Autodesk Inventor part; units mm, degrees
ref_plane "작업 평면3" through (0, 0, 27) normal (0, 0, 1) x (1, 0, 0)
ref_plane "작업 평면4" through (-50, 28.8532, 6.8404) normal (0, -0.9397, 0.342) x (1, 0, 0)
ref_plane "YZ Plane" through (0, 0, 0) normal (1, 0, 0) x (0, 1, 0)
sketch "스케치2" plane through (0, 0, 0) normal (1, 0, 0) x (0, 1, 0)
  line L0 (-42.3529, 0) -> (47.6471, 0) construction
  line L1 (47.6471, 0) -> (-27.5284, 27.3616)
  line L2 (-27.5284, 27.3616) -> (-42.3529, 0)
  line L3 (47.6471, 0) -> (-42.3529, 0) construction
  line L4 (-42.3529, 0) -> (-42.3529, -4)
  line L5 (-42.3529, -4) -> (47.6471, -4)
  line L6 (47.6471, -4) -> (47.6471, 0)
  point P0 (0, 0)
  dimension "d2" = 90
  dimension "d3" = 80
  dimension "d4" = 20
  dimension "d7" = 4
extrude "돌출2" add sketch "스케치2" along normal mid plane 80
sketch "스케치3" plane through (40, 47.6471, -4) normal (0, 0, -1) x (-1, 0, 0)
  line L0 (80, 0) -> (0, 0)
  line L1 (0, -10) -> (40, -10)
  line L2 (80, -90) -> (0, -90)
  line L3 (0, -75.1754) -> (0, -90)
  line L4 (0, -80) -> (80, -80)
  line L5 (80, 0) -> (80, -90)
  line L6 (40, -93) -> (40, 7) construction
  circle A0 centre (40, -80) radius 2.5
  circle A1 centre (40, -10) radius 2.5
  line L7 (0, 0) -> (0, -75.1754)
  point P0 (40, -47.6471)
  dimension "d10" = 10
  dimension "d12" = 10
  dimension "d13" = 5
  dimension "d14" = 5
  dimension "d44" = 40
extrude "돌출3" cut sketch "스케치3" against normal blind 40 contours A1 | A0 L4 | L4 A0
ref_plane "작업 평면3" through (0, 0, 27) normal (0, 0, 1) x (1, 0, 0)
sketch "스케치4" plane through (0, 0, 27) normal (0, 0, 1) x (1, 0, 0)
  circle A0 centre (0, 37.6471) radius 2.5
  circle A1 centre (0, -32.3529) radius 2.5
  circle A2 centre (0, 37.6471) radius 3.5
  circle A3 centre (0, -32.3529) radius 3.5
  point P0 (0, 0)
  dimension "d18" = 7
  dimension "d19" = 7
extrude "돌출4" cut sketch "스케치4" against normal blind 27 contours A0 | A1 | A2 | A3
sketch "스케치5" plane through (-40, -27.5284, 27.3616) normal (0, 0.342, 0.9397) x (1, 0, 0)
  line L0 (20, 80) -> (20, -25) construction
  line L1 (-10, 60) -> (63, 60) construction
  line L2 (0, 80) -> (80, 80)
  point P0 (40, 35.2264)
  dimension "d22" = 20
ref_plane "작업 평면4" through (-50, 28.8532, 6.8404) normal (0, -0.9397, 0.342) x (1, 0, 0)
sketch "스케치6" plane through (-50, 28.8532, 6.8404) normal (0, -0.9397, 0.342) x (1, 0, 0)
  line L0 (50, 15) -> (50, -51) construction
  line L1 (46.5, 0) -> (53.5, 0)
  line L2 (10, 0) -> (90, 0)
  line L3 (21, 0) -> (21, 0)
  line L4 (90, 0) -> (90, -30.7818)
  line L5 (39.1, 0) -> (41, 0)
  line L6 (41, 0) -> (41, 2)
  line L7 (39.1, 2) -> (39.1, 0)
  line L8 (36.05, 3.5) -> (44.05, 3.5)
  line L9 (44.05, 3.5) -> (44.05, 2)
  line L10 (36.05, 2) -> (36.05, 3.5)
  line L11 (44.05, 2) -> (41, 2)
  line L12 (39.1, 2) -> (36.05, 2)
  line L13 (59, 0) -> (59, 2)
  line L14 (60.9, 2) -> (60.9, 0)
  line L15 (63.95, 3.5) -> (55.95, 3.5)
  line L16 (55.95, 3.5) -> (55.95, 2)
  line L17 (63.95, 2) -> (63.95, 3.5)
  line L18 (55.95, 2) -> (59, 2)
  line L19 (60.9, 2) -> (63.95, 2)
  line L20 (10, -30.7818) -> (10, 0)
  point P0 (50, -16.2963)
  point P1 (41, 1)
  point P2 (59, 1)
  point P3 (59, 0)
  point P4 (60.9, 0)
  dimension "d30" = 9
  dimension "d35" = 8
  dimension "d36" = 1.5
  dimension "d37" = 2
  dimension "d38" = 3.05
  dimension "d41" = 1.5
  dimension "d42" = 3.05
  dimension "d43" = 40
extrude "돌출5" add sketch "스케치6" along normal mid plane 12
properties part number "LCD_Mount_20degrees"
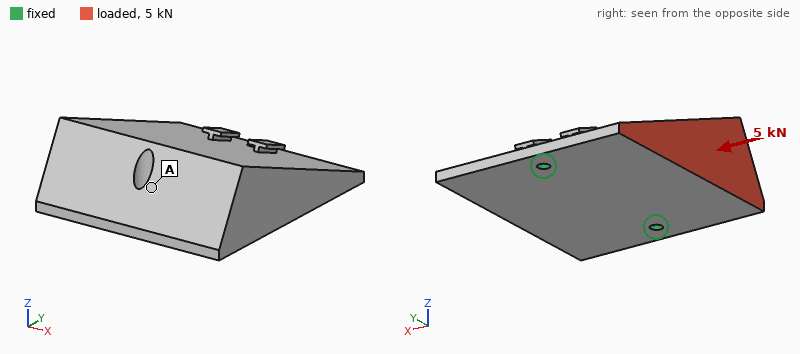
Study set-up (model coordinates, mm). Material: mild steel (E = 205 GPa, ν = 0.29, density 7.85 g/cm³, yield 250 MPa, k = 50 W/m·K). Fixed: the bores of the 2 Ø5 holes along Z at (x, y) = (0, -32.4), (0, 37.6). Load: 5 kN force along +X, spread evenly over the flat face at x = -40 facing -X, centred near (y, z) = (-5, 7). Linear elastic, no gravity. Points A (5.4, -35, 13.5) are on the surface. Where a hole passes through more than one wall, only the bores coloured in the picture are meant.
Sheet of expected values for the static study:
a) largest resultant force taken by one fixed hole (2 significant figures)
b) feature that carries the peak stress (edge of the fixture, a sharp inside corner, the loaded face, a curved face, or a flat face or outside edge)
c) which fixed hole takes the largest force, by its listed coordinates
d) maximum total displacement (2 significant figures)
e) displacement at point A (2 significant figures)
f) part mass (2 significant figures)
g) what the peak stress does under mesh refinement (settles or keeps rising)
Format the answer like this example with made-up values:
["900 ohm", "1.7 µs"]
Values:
["3.0 kN", "edge of the fixture", "(0, -32.4)", "69 µm", "24 µm", "990 g", "keeps rising"]
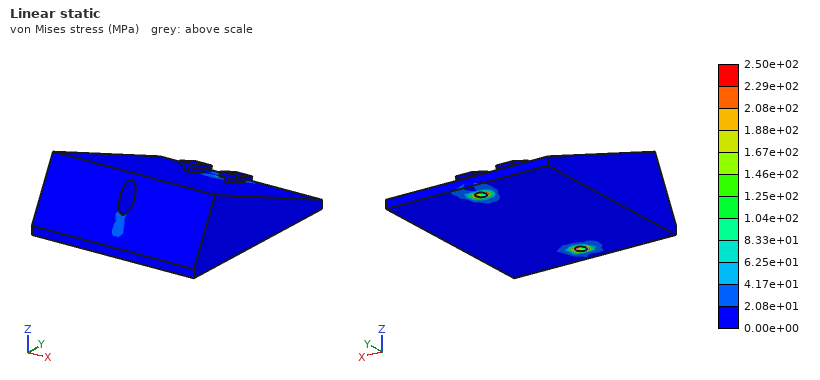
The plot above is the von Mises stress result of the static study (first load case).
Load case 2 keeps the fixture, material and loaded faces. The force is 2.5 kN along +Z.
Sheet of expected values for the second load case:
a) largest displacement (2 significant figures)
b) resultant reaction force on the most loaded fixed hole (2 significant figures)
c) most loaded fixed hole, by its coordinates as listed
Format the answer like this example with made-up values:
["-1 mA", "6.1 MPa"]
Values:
["0.16 mm", "1.8 kN", "(0, -32.4)"]
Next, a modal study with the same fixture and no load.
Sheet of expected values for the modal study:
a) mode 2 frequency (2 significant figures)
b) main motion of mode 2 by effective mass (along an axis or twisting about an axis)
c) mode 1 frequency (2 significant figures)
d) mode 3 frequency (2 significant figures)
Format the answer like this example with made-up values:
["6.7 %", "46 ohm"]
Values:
["5000 Hz", "along Z", "1100 Hz", "8000 Hz"]
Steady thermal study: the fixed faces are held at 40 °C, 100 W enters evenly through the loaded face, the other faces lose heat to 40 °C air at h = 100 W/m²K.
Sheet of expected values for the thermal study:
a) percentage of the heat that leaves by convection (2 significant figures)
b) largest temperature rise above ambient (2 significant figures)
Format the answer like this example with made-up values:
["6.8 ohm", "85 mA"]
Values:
["55 %", "67 K"]
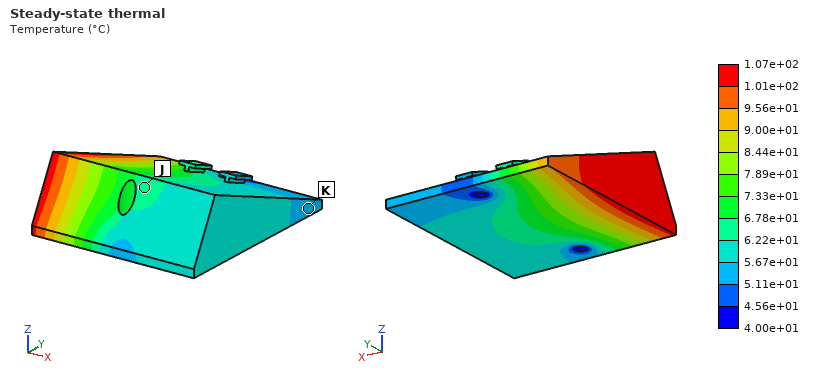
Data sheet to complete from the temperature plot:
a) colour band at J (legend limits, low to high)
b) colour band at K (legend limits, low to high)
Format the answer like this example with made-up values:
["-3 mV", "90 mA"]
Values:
["6.22e+01 to 6.78e+01 °C", "5.11e+01 to 5.67e+01 °C"]
